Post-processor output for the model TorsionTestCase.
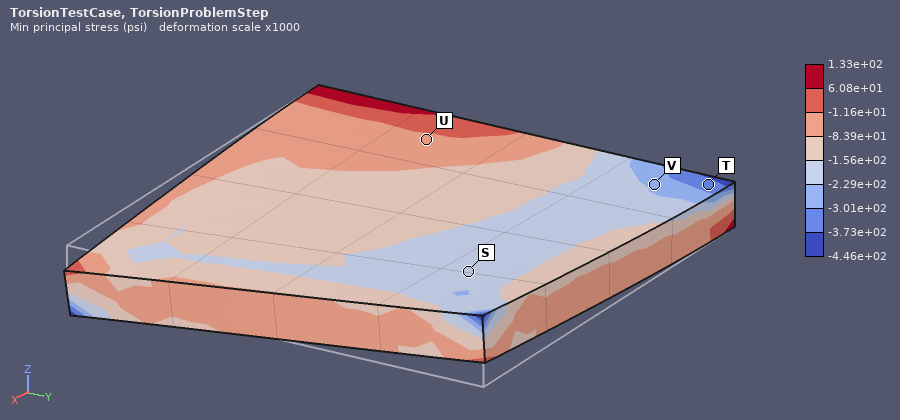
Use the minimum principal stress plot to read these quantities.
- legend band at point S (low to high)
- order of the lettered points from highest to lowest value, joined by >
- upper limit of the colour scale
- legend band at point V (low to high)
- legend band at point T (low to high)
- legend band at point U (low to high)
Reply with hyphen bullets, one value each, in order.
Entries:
- -2.29e+02 to -1.56e+02 psi
- U > S > V > T
- 1.33e+02 psi
- -3.01e+02 to -2.29e+02 psi
- -3.73e+02 to -3.01e+02 psi
- -8.39e+01 to -1.16e+01 psi
